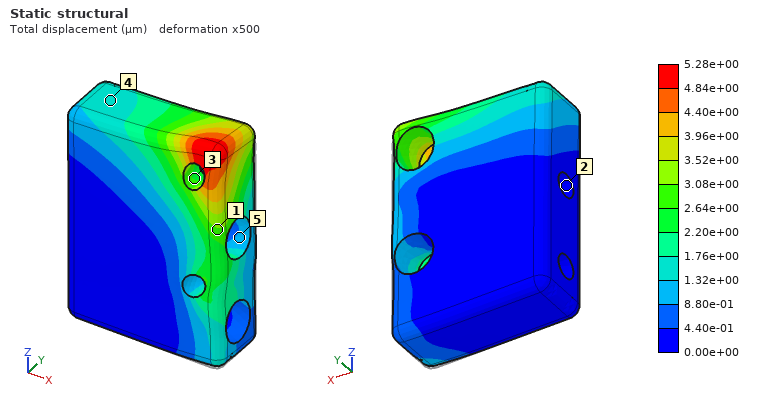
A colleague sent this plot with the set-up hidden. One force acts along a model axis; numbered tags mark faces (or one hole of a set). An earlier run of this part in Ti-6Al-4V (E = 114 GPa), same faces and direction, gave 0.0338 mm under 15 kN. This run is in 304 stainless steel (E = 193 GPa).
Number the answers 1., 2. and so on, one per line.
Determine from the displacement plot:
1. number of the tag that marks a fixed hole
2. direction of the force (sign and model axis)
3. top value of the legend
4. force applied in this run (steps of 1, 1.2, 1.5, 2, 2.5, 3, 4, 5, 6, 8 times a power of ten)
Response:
1. 2
2. +Z
3. 5.28e+00 µm
4. 4 kN
